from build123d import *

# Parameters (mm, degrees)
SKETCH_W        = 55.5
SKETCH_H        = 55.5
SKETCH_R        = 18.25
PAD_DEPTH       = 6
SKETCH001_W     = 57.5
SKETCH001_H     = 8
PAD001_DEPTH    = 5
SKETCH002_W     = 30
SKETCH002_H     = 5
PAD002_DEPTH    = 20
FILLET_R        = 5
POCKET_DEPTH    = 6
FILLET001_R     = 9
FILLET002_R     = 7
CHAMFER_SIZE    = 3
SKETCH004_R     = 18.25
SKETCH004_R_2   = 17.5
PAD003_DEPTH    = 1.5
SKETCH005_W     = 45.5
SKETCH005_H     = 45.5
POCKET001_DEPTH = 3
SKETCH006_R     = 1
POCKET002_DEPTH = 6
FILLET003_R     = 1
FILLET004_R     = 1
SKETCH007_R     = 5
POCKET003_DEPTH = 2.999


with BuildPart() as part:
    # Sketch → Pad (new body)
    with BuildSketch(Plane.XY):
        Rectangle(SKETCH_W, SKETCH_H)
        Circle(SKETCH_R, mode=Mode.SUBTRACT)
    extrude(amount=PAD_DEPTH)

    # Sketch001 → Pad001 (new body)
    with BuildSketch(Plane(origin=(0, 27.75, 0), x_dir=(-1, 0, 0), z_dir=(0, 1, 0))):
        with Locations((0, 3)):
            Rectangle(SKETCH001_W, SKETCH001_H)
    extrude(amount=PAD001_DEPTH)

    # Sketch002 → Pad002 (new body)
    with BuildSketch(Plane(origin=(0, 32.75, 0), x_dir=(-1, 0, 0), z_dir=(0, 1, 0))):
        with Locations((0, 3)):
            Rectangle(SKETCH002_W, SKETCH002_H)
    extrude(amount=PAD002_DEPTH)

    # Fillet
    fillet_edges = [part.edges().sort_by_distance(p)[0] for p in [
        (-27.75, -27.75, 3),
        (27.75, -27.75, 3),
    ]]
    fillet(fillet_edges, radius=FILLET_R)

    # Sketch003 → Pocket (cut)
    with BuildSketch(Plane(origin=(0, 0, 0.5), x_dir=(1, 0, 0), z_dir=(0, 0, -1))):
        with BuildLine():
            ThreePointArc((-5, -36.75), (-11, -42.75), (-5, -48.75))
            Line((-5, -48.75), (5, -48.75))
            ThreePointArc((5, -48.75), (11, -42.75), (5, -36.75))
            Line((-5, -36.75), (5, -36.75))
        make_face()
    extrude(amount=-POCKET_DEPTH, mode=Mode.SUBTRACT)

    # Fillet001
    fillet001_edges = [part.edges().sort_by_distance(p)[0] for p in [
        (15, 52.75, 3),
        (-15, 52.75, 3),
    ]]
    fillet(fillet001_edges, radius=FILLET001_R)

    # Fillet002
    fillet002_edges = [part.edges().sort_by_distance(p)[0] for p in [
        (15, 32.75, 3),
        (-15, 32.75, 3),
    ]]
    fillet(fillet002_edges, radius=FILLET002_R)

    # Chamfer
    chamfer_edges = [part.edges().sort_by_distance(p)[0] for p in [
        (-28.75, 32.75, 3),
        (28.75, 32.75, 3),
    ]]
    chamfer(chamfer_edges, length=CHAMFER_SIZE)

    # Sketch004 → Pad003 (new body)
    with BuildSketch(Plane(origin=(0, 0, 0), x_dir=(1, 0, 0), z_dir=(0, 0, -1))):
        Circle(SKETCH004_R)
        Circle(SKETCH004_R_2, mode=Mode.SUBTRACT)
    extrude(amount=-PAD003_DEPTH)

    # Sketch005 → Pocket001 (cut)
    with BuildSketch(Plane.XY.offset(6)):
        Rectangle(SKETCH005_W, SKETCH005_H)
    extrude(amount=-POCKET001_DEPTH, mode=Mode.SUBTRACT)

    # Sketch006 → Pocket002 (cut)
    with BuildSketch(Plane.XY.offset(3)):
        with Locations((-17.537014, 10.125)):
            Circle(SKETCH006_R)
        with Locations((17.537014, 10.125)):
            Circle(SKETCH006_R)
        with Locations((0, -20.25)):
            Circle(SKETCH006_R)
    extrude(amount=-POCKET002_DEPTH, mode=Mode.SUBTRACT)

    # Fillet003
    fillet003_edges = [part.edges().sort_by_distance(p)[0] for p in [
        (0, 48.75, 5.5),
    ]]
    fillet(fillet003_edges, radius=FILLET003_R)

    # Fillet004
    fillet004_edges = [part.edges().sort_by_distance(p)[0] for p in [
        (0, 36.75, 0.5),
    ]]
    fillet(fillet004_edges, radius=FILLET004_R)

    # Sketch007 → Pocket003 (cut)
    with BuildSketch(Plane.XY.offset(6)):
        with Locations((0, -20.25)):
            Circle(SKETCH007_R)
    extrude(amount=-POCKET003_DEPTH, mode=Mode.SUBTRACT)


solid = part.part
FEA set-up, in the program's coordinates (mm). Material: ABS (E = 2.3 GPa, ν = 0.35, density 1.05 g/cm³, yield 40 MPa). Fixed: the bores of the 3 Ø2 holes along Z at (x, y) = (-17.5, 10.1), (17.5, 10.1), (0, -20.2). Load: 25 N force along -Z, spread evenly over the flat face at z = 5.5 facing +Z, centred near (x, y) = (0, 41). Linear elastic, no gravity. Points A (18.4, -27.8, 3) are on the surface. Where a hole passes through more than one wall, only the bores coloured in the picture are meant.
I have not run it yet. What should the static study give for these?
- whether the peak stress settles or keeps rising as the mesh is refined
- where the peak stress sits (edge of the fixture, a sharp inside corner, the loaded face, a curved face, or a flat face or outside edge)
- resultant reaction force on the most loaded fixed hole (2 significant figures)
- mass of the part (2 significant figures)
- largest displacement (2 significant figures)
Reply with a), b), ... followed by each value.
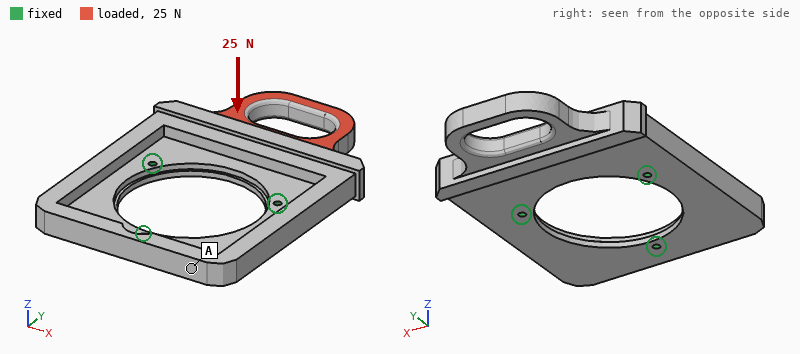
a) keeps rising
b) edge of the fixture
c) 20 N
d) 14 g
e) 1.1 mm
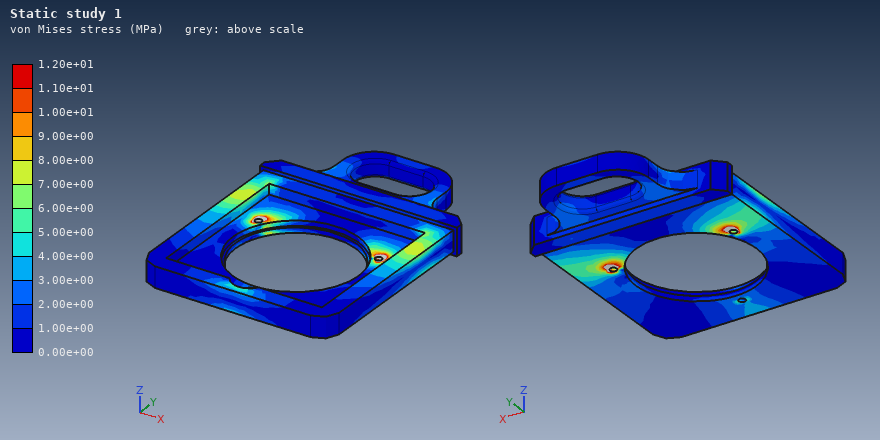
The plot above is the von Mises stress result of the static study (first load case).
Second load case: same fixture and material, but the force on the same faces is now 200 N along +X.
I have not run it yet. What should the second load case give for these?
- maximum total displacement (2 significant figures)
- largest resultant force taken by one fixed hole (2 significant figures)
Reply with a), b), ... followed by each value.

a) 0.33 mm
b) 180 N
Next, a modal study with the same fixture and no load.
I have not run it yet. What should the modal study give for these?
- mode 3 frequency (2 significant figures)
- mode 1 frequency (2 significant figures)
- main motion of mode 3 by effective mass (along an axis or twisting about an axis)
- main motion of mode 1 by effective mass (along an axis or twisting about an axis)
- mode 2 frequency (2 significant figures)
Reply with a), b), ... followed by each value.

a) 1500 Hz
b) 530 Hz
c) along Z
d) along Z
e) 1000 Hz
